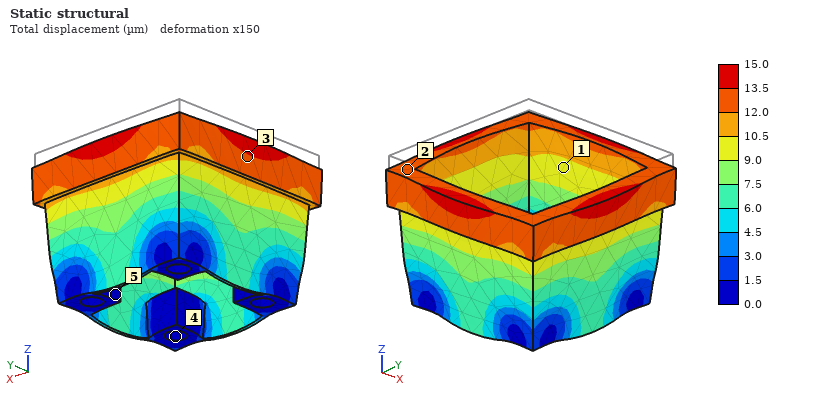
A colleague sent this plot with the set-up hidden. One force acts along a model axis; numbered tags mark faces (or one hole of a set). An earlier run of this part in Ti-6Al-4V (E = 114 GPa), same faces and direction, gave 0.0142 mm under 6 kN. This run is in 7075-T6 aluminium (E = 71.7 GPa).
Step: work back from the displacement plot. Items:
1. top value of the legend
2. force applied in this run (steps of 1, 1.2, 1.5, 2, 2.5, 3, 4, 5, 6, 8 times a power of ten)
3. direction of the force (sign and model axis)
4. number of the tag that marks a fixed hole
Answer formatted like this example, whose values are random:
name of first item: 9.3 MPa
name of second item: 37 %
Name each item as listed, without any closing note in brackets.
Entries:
top value of the legend: 15.0 µm
force applied in this run: 4 kN
direction of the force: -Z
number of the tag that marks a fixed hole: 4
